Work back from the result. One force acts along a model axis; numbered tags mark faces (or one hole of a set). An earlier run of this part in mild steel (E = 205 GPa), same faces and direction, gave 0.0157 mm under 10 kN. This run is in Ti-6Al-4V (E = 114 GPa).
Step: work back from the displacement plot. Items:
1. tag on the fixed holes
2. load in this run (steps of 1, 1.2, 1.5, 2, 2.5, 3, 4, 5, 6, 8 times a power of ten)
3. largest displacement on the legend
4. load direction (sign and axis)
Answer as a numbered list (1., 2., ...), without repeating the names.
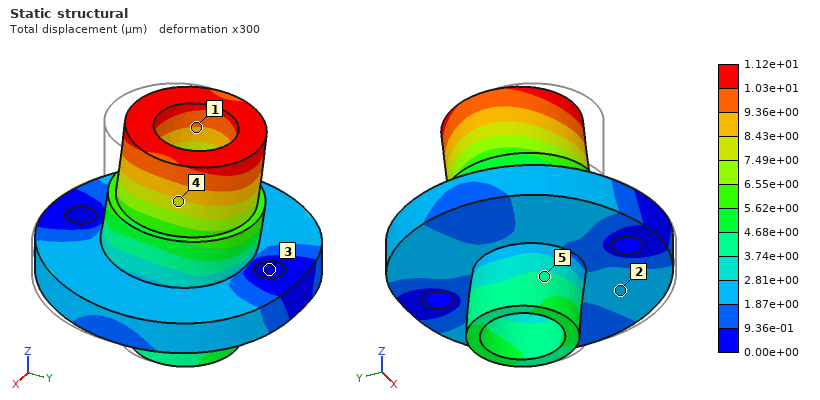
1. 3
2. 4 kN
3. 1.12e+01 µm
4. +Y
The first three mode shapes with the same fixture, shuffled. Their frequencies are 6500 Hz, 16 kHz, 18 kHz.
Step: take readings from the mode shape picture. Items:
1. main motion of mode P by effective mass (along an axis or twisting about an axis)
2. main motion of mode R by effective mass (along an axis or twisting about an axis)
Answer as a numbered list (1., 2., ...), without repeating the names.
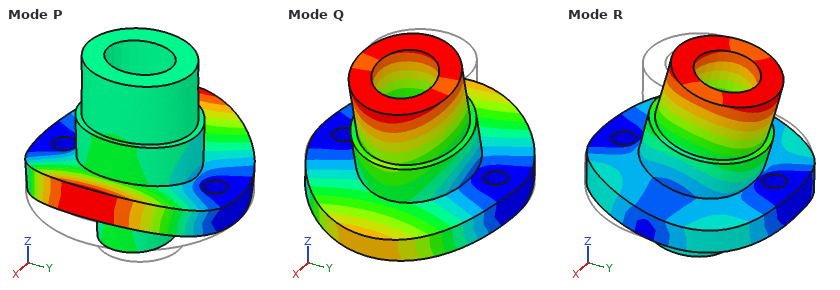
1. along Z
2. along Y
